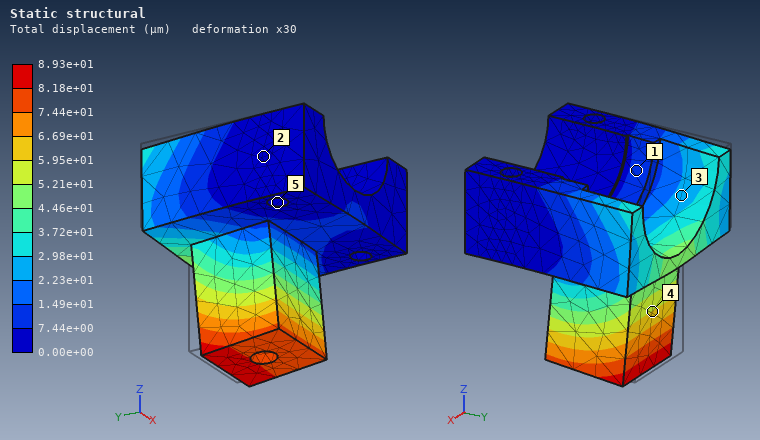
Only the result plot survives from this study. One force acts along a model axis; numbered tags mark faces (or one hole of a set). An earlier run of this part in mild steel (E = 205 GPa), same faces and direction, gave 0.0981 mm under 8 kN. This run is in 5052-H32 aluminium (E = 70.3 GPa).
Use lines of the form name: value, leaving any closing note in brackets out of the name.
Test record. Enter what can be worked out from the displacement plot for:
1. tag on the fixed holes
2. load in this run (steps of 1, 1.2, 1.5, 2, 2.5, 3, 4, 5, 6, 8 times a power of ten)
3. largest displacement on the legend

tag on the fixed holes: 5
load in this run: 2.5 kN
largest displacement on the legend: 8.93e+01 µm
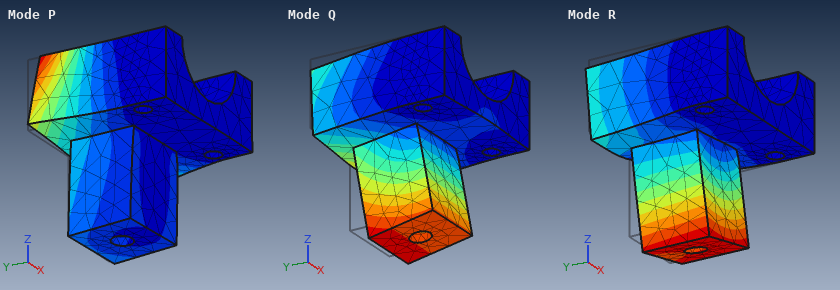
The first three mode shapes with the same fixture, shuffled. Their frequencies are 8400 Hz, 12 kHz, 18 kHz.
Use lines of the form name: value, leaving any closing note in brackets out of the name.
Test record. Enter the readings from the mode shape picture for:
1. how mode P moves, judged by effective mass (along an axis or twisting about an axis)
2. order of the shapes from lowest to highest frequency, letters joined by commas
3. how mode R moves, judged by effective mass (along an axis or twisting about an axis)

how mode P moves, judged by effective mass: along X
order of the shapes from lowest to highest frequency, letters joined by commas: Q, R, P
how mode R moves, judged by effective mass: along X
